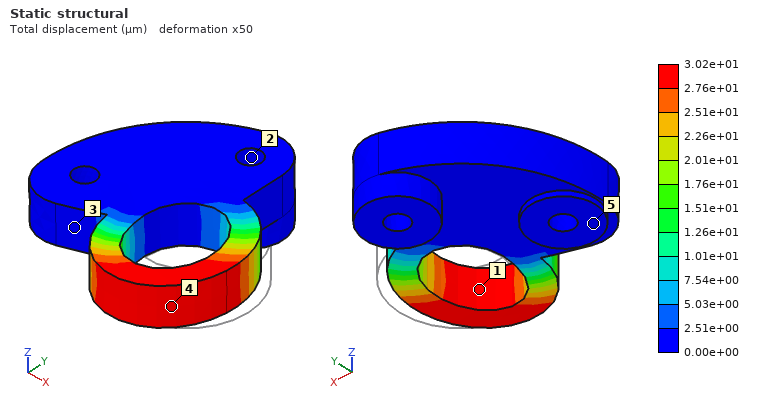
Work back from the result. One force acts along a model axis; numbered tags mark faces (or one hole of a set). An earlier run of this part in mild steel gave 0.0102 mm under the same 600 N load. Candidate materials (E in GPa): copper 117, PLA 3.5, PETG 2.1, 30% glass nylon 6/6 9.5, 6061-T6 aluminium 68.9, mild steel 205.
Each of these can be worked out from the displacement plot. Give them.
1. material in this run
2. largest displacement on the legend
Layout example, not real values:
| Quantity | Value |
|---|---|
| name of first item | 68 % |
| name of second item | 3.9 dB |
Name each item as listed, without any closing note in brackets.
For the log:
| Quantity | Value |
|---|---|
| material in this run | 6061-T6 aluminium |
| largest displacement on the legend | 3.02e+01 µm |
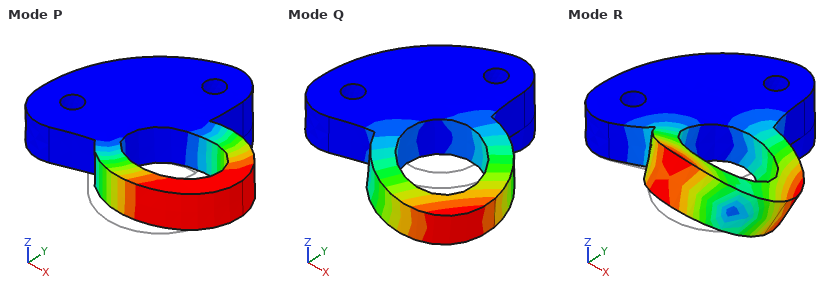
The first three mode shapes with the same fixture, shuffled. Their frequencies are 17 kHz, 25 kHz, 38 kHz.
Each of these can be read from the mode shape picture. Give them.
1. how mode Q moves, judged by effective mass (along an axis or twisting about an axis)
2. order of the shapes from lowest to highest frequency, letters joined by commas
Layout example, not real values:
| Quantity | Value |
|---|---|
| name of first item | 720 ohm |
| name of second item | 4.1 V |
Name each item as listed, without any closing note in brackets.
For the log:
| Quantity | Value |
|---|---|
| how mode Q moves, judged by effective mass | along Z |
| order of the shapes from lowest to highest frequency, letters joined by commas | Q, P, R |
